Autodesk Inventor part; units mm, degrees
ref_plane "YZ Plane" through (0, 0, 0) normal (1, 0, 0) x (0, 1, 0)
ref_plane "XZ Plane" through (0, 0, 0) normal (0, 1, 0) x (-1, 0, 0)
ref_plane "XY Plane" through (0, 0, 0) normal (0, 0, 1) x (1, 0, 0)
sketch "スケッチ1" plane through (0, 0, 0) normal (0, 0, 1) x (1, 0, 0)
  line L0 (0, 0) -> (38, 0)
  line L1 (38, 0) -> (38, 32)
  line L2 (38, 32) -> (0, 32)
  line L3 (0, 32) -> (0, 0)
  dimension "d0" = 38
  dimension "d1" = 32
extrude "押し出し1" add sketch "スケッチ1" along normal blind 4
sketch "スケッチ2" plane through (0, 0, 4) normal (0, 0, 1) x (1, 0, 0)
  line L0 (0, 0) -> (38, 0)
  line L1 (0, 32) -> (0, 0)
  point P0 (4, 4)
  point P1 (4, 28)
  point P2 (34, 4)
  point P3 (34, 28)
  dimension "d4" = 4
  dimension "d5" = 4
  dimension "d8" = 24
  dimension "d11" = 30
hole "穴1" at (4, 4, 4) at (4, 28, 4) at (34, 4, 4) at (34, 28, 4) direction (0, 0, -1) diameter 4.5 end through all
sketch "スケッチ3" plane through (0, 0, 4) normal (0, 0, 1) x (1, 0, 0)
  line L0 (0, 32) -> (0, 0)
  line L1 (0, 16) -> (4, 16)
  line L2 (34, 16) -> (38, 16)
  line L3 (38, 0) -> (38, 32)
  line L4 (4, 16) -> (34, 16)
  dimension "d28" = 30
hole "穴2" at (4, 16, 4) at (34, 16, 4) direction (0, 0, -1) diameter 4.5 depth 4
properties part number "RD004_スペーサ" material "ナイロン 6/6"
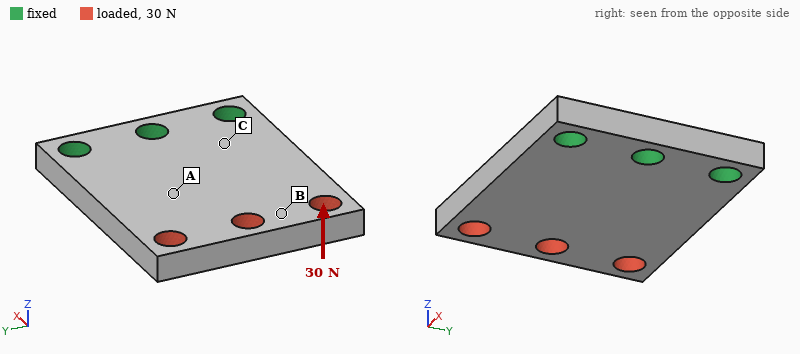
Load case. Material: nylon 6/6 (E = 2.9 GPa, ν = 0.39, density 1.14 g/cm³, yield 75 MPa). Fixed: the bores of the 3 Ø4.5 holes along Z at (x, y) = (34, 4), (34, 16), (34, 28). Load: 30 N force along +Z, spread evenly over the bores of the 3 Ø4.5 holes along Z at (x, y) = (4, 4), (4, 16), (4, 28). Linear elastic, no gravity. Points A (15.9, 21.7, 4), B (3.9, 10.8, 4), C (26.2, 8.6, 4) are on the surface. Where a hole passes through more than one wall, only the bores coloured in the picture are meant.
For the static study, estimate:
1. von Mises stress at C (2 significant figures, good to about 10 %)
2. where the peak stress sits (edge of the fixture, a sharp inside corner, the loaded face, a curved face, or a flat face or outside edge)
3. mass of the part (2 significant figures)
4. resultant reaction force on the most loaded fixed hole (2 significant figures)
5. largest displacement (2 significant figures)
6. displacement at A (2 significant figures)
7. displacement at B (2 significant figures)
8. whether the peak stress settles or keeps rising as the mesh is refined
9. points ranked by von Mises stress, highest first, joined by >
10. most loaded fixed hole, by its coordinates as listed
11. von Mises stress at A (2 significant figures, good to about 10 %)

6.9 MPa
edge of the fixture
5.1 g
21 N
0.56 mm
0.20 mm
0.46 mm
keeps rising
C > A > B
(34, 16)
3.9 MPa
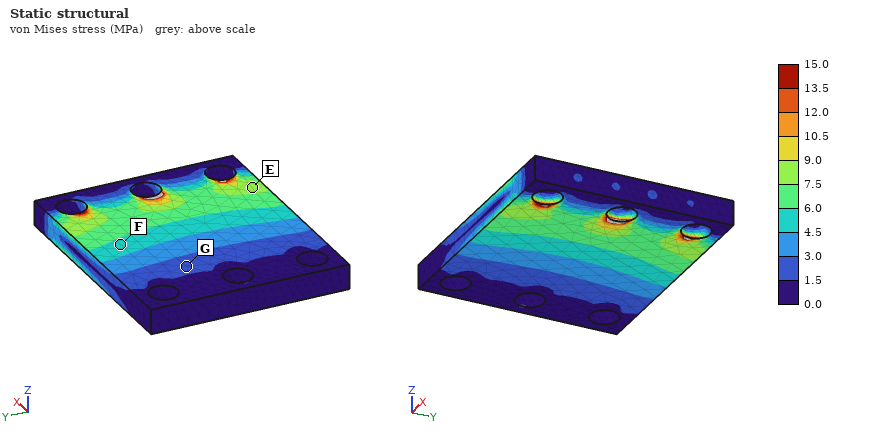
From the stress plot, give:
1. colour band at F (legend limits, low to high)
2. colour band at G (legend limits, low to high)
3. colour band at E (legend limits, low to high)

4.5 to 6.0 MPa
1.5 to 3.0 MPa
7.5 to 9.0 MPa
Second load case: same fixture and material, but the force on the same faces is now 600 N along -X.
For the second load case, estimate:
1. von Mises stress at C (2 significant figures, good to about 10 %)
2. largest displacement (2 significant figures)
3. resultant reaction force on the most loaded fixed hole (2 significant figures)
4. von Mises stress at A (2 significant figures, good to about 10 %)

4.1 MPa
70 µm
200 N
4.5 MPa
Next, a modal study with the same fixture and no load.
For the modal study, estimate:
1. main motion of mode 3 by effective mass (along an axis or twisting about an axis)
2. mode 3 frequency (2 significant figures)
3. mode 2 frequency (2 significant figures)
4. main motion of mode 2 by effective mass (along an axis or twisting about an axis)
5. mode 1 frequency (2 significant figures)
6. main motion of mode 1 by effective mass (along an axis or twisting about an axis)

along Y
5200 Hz
2400 Hz
twisting about X
1100 Hz
along Z
